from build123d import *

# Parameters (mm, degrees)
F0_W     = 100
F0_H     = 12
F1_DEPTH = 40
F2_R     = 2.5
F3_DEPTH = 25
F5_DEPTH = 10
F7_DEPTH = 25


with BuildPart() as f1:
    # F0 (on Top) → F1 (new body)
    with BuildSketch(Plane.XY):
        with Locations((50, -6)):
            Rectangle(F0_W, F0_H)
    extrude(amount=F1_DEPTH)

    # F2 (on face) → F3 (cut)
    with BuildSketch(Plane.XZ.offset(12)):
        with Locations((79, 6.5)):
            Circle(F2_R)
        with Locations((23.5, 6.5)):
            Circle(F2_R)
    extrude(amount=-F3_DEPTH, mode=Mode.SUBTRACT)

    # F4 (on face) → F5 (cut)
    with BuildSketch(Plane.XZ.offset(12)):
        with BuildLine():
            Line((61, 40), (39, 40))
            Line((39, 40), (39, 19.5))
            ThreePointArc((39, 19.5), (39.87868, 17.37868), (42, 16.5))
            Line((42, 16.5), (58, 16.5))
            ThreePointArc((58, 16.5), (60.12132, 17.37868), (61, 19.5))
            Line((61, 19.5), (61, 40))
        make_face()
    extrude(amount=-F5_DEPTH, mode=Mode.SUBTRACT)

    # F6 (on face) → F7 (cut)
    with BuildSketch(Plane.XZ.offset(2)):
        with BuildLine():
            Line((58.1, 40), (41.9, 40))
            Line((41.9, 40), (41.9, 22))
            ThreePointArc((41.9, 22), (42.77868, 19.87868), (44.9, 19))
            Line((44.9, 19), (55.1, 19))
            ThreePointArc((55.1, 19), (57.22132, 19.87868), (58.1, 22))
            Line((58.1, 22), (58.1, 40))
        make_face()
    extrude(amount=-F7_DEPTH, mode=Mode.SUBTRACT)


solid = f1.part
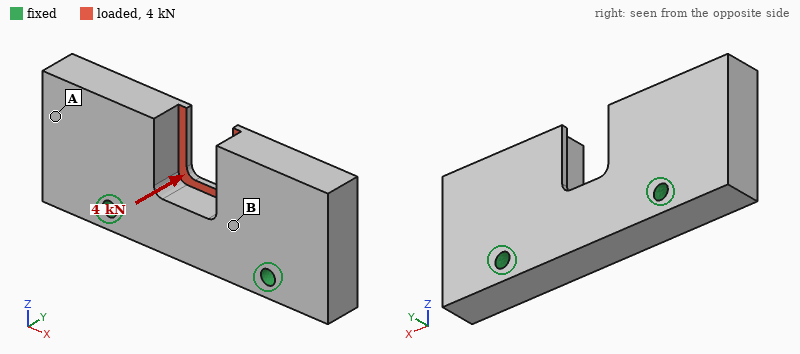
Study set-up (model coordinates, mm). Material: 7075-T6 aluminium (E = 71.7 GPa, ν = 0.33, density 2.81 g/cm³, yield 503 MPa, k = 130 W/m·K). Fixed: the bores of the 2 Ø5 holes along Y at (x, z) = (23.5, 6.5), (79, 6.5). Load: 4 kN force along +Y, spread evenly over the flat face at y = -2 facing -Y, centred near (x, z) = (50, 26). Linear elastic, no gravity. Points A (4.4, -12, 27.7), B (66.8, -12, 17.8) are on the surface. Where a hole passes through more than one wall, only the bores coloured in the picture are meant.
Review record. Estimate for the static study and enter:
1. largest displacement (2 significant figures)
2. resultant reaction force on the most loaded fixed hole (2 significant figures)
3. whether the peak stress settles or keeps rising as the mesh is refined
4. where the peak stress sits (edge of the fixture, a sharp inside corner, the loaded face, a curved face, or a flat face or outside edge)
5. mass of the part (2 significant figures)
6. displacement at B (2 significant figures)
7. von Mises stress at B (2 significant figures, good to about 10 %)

0.11 mm
2.1 kN
keeps rising
edge of the fixture
120 g
0.031 mm
36 MPa
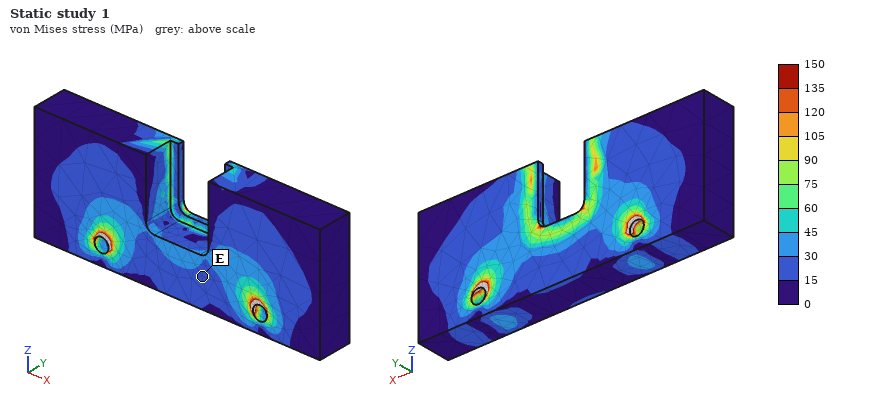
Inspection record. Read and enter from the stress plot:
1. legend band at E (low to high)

15 to 30 MPa
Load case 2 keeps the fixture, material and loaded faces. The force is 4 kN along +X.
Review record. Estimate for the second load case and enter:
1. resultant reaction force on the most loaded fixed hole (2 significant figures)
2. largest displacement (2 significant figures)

2.3 kN
21 µm
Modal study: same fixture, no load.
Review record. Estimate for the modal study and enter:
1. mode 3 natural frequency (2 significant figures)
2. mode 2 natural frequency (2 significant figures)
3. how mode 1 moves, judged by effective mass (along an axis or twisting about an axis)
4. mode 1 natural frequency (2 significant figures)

6800 Hz
6500 Hz
along Y
6100 Hz
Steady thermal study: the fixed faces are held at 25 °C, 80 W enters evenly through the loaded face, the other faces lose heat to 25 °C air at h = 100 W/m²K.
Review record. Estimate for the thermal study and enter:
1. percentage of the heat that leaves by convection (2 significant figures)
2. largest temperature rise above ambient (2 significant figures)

14 %
40 K
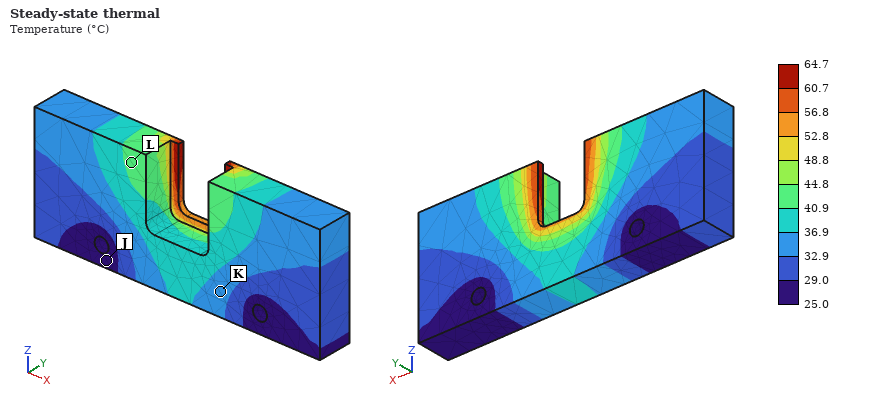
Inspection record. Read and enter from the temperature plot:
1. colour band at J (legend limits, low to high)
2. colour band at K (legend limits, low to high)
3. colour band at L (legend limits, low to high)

25.0 to 29.0 °C
32.9 to 36.9 °C
40.9 to 44.8 °C
